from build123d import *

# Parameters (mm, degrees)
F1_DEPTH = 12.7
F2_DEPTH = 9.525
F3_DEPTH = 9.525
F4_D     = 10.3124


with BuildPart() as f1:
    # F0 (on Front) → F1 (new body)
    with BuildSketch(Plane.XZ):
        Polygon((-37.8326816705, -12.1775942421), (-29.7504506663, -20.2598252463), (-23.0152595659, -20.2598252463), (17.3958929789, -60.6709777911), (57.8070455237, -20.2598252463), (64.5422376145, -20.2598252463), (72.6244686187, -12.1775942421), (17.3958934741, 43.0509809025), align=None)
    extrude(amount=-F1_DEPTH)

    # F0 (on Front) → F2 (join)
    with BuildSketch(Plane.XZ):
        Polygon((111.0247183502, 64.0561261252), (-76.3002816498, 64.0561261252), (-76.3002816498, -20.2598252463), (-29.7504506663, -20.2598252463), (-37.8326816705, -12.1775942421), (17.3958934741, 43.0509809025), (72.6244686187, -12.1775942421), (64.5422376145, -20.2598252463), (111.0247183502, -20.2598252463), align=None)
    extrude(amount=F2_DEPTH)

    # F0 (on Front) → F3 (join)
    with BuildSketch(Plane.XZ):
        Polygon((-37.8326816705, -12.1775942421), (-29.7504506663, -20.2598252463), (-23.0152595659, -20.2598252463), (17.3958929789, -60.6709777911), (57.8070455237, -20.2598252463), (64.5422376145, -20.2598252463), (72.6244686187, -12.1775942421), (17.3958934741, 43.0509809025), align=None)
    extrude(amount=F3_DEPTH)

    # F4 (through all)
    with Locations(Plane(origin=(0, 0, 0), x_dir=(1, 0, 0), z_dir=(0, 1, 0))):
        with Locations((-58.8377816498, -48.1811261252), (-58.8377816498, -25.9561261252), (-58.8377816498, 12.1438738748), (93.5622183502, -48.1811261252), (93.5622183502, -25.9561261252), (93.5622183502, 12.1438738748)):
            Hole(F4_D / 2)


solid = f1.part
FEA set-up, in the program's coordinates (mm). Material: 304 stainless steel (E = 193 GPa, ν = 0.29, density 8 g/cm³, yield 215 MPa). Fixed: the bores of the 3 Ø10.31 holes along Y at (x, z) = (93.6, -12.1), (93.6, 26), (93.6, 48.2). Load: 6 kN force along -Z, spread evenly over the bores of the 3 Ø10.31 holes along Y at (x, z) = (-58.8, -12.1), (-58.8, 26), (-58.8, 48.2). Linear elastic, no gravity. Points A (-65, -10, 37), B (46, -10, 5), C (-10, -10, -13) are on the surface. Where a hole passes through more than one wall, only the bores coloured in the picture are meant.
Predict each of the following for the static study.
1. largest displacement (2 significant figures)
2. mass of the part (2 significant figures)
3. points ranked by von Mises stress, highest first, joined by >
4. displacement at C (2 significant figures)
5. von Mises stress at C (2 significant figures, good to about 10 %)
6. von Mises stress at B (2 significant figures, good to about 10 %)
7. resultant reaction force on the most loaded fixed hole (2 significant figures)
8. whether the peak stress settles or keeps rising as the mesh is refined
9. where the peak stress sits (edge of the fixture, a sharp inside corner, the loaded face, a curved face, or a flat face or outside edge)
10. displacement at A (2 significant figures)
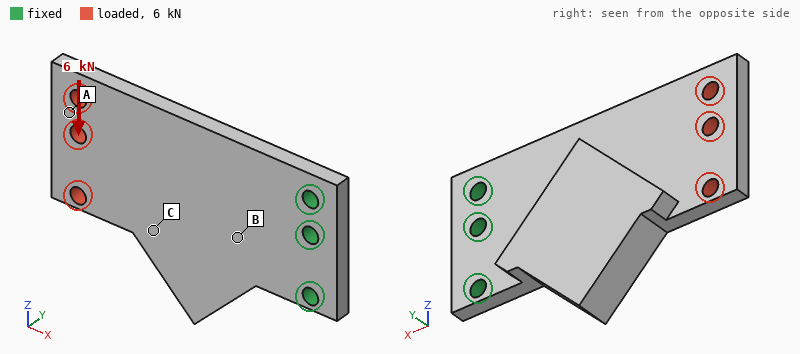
0.12 mm
1.8 kg
B > C > A
0.055 mm
18 MPa
34 MPa
14 kN
keeps rising
edge of the fixture
0.10 mm
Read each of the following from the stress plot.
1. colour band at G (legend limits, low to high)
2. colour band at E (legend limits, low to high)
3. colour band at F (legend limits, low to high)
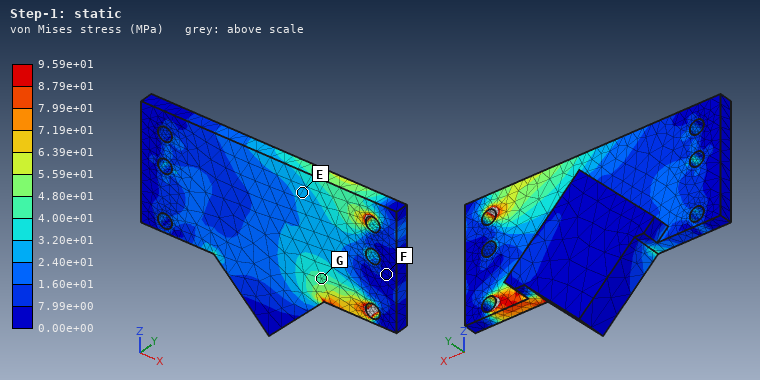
4.00e+01 to 4.80e+01 MPa
2.40e+01 to 3.20e+01 MPa
0.00e+00 to 7.99e+00 MPa
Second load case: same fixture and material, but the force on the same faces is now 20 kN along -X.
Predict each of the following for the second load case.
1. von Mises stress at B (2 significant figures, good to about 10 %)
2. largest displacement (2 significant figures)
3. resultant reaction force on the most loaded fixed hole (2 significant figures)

26 MPa
57 µm
6.9 kN
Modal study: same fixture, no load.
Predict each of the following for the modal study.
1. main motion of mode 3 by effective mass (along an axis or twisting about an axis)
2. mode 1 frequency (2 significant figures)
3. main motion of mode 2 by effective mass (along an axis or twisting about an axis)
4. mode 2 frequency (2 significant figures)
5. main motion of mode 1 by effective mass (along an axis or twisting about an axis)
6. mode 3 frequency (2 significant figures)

along Z
290 Hz
twisting about X
1200 Hz
along Y
1800 Hz
